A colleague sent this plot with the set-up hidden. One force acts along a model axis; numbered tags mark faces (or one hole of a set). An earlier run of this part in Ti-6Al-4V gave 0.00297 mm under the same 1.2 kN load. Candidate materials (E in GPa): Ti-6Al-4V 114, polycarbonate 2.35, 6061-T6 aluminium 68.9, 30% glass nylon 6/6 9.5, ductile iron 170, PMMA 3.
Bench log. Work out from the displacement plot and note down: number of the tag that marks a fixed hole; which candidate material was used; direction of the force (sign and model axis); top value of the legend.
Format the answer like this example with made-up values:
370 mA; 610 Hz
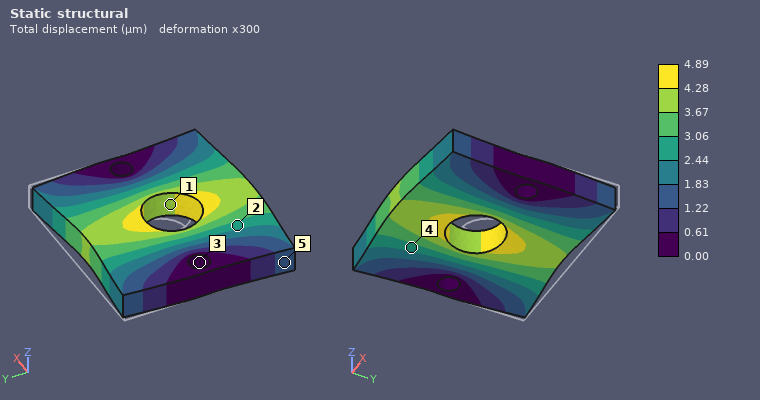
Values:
3; 6061-T6 aluminium; -Y; 4.89 µm
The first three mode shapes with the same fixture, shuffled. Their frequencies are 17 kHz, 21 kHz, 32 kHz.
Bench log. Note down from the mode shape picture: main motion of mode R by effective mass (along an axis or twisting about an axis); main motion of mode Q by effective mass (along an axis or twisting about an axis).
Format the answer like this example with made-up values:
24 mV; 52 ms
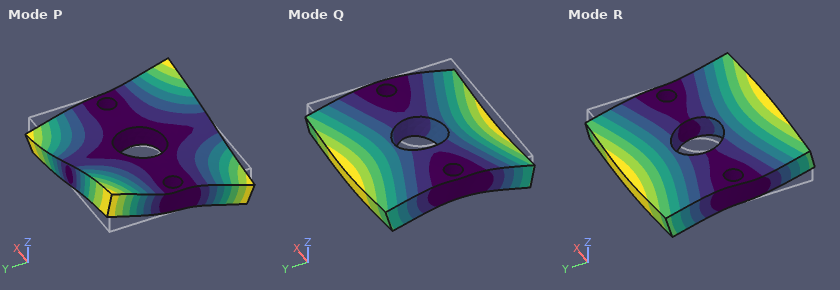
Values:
twisting about X; along Z
